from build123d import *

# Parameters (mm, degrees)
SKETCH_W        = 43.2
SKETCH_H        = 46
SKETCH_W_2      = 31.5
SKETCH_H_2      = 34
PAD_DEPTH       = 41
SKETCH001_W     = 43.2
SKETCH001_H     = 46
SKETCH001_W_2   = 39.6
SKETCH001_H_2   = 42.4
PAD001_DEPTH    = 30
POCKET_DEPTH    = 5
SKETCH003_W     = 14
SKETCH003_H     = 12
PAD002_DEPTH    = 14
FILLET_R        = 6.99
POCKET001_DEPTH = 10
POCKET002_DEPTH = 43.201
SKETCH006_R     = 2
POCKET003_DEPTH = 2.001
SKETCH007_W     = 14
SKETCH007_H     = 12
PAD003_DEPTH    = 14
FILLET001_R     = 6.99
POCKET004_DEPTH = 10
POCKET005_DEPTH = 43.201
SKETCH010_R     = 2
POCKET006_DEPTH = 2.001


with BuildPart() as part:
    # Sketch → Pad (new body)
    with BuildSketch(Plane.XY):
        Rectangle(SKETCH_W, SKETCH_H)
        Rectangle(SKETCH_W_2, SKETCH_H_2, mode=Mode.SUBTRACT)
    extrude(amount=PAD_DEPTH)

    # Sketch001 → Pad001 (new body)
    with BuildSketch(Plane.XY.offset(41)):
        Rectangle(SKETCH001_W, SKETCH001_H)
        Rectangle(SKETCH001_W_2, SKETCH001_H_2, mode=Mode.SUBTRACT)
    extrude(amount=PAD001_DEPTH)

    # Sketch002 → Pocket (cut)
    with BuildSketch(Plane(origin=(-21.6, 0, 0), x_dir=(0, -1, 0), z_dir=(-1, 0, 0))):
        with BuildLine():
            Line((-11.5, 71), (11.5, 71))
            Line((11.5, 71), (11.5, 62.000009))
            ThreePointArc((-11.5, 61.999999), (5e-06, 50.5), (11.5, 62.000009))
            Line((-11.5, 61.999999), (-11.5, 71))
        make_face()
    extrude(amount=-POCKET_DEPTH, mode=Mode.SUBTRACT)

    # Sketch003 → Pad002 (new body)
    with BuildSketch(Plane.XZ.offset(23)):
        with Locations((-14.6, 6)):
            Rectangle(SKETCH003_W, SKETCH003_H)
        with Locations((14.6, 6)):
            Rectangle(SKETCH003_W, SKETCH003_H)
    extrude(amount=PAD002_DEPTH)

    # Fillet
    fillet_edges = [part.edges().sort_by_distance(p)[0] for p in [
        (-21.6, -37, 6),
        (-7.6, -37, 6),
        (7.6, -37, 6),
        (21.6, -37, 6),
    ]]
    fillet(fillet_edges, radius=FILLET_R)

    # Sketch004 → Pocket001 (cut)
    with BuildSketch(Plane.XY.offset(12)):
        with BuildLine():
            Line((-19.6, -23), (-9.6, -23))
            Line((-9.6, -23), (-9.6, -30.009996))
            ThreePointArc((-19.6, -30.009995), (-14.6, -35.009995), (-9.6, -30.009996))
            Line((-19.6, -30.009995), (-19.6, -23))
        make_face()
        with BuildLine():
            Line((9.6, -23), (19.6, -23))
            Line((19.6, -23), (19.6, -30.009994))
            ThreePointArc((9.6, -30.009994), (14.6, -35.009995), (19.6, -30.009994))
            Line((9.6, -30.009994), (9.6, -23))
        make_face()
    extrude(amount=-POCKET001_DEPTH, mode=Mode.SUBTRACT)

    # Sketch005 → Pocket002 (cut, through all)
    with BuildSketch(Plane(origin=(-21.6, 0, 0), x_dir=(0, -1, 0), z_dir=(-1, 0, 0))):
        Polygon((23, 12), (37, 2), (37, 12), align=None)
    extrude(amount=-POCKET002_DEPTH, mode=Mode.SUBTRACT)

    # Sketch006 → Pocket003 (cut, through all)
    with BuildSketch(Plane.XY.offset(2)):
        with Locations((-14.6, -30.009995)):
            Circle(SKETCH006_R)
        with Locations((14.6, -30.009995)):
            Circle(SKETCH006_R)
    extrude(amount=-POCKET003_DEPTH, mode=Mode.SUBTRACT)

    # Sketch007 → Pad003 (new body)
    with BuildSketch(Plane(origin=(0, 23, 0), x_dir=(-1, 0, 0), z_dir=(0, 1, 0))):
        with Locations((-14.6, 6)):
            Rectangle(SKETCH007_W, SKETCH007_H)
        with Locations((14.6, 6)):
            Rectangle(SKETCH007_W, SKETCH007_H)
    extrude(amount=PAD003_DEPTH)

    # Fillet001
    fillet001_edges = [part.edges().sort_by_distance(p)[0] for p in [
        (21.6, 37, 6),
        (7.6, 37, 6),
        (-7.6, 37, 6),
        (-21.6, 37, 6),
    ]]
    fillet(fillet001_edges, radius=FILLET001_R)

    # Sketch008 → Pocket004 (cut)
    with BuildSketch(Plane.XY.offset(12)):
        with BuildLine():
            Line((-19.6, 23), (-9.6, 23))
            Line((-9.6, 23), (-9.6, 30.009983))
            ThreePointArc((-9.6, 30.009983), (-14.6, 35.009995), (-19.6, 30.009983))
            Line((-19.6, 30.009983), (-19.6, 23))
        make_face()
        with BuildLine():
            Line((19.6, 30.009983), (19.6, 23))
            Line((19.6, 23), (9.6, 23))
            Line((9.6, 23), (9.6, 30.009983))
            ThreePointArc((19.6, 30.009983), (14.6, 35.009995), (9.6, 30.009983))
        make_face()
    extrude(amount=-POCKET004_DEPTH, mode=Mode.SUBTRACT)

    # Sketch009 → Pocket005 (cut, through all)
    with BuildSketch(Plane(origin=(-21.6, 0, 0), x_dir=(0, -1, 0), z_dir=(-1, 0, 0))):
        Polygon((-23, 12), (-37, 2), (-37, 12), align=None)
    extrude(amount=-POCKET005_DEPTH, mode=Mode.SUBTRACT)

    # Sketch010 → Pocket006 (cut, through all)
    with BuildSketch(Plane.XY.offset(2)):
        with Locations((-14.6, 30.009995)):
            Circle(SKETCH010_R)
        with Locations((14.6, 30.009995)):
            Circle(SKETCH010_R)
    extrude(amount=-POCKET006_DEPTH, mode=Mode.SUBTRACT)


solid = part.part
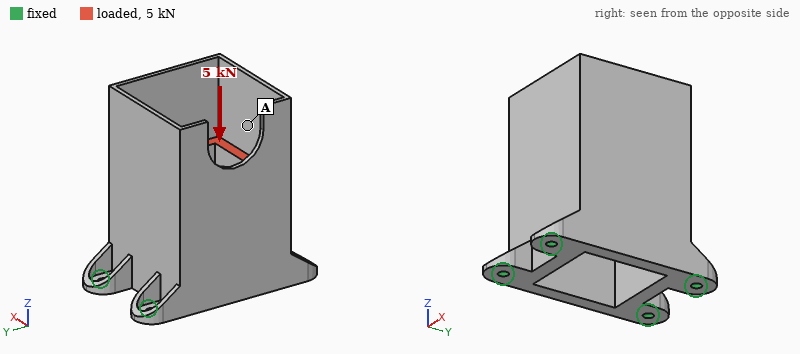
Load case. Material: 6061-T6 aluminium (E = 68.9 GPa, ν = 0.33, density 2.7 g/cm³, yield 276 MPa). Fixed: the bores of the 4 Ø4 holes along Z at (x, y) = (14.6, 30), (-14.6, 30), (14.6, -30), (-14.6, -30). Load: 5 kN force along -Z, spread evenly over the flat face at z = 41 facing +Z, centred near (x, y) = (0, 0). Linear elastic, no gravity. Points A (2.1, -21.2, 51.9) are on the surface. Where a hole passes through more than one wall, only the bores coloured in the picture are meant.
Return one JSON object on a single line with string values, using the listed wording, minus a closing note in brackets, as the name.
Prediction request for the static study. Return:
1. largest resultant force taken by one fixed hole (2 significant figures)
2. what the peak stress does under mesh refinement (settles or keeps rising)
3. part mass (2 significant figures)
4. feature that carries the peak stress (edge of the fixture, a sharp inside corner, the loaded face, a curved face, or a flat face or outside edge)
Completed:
{"largest resultant force taken by one fixed hole": "1.4 kN", "what the peak stress does under mesh refinement": "keeps rising", "part mass": "130 g", "feature that carries the peak stress": "edge of the fixture"}
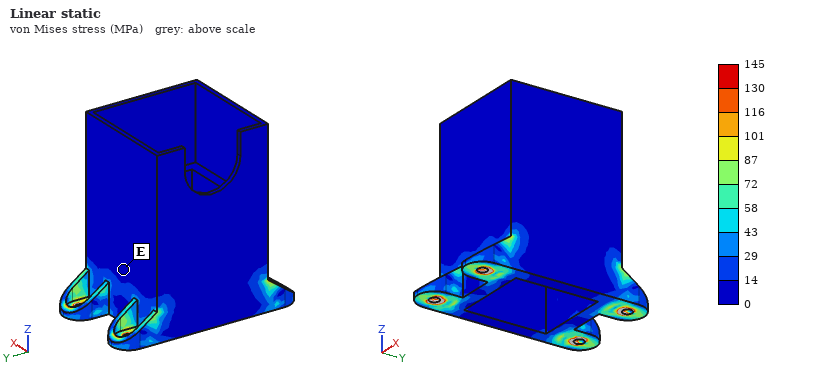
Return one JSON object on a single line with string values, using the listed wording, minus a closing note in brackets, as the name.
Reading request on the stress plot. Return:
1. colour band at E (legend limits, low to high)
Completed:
{"colour band at E": "0 to 14 MPa"}
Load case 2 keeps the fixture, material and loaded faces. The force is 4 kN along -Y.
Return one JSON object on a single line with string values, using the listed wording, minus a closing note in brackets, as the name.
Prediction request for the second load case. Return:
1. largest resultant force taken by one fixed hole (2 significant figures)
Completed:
{"largest resultant force taken by one fixed hole": "1.7 kN"}
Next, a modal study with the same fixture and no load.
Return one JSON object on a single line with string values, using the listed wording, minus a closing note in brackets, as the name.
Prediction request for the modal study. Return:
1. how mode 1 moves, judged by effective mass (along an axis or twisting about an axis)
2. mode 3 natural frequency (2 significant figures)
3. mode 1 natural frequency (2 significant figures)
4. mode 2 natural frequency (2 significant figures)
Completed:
{"how mode 1 moves, judged by effective mass": "along X", "mode 3 natural frequency": "3800 Hz", "mode 1 natural frequency": "2200 Hz", "mode 2 natural frequency": "3700 Hz"}
